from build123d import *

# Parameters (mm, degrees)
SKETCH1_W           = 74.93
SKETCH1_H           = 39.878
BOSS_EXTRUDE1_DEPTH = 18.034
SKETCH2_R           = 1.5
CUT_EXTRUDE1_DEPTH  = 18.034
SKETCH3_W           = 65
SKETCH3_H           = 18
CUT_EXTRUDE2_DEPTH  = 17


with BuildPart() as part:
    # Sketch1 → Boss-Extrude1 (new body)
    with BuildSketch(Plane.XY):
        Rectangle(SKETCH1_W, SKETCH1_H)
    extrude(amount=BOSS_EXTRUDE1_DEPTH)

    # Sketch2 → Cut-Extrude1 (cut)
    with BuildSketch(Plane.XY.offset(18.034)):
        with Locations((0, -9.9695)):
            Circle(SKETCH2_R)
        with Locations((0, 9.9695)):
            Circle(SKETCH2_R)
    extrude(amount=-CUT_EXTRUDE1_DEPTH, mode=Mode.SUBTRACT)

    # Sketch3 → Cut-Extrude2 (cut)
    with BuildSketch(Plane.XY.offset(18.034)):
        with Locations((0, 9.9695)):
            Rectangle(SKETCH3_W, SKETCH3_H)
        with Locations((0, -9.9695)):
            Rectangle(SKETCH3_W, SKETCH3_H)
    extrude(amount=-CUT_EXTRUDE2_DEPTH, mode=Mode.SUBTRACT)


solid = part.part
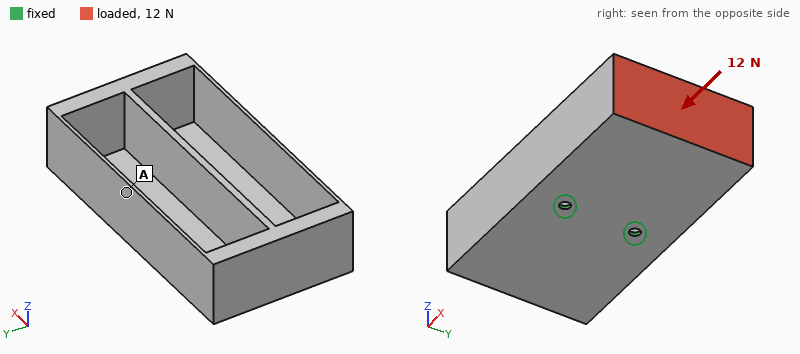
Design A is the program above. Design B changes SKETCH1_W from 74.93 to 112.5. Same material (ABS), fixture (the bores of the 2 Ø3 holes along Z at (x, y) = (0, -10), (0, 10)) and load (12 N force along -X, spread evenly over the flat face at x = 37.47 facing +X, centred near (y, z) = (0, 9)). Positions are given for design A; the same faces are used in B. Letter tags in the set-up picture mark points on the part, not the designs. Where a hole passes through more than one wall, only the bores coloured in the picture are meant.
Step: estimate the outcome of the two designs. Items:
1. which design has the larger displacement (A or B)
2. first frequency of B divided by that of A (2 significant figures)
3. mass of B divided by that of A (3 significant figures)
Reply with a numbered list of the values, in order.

1. B
2. 0.41
3. 2.92
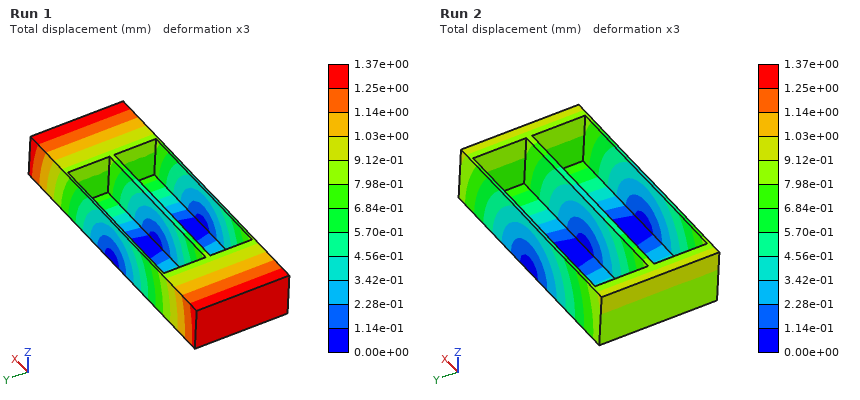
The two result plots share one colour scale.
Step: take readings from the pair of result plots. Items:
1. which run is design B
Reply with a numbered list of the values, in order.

1. Run 1
